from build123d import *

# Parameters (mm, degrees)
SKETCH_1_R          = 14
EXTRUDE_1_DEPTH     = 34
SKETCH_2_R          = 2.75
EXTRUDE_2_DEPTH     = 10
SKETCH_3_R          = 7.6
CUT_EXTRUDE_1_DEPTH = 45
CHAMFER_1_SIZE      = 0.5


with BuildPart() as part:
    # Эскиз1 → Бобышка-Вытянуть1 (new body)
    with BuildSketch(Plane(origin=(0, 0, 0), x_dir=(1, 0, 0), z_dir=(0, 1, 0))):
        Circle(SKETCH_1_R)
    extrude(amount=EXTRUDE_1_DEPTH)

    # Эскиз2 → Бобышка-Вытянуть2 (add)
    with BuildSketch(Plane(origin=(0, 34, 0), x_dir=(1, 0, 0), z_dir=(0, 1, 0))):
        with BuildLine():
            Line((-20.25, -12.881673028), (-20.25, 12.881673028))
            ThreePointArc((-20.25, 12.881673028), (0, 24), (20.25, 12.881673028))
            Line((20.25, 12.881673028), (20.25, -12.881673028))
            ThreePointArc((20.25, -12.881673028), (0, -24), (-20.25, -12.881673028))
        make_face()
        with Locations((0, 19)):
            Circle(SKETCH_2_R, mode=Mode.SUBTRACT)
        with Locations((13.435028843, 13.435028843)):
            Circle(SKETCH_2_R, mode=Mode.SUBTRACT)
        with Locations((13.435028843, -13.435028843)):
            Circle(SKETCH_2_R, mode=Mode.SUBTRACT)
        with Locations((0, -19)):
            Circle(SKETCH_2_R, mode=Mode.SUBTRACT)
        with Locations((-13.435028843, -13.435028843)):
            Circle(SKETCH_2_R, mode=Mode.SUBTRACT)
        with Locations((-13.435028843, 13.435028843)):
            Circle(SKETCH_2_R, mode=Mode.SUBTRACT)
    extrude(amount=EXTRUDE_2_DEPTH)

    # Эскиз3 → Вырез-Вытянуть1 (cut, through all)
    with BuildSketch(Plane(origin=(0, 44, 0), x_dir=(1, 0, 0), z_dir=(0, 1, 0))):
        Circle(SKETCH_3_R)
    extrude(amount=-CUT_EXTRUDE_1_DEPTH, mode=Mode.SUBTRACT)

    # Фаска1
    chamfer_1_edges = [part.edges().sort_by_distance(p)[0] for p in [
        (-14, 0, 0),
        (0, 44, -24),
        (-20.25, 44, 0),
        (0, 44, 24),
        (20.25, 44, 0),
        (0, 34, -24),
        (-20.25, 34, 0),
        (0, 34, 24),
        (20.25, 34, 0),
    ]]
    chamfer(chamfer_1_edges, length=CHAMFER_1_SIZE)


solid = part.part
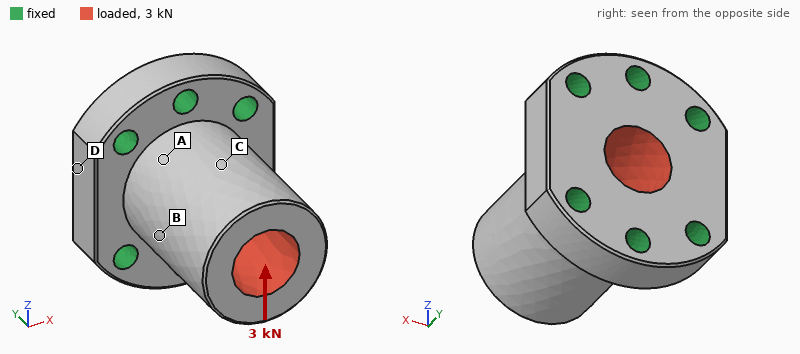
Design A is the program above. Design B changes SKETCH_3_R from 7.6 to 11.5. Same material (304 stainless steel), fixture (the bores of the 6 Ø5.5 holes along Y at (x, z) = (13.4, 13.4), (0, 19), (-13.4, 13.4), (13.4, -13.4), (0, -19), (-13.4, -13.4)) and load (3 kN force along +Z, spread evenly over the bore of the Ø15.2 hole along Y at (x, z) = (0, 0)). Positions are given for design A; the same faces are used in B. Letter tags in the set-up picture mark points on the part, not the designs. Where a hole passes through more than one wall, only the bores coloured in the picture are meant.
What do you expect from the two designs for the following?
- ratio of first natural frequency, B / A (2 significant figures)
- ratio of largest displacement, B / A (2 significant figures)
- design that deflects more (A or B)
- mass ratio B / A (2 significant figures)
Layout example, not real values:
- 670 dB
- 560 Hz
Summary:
- 1.1
- 1.8
- B
- 0.64
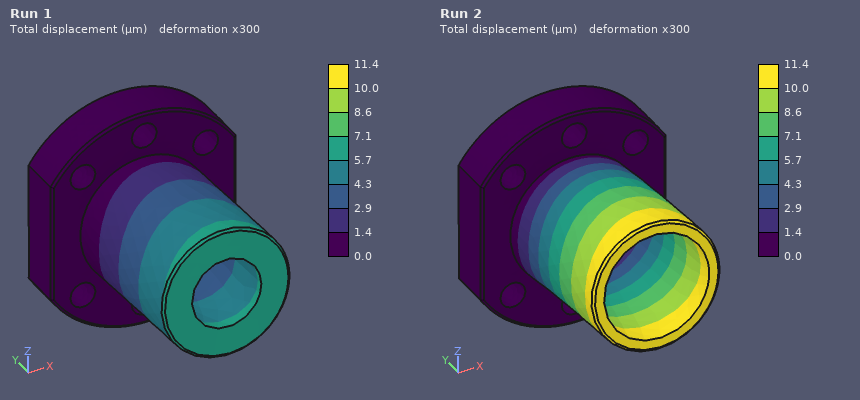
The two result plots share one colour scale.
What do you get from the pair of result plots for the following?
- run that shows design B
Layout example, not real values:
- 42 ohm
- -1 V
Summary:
- Run 2
